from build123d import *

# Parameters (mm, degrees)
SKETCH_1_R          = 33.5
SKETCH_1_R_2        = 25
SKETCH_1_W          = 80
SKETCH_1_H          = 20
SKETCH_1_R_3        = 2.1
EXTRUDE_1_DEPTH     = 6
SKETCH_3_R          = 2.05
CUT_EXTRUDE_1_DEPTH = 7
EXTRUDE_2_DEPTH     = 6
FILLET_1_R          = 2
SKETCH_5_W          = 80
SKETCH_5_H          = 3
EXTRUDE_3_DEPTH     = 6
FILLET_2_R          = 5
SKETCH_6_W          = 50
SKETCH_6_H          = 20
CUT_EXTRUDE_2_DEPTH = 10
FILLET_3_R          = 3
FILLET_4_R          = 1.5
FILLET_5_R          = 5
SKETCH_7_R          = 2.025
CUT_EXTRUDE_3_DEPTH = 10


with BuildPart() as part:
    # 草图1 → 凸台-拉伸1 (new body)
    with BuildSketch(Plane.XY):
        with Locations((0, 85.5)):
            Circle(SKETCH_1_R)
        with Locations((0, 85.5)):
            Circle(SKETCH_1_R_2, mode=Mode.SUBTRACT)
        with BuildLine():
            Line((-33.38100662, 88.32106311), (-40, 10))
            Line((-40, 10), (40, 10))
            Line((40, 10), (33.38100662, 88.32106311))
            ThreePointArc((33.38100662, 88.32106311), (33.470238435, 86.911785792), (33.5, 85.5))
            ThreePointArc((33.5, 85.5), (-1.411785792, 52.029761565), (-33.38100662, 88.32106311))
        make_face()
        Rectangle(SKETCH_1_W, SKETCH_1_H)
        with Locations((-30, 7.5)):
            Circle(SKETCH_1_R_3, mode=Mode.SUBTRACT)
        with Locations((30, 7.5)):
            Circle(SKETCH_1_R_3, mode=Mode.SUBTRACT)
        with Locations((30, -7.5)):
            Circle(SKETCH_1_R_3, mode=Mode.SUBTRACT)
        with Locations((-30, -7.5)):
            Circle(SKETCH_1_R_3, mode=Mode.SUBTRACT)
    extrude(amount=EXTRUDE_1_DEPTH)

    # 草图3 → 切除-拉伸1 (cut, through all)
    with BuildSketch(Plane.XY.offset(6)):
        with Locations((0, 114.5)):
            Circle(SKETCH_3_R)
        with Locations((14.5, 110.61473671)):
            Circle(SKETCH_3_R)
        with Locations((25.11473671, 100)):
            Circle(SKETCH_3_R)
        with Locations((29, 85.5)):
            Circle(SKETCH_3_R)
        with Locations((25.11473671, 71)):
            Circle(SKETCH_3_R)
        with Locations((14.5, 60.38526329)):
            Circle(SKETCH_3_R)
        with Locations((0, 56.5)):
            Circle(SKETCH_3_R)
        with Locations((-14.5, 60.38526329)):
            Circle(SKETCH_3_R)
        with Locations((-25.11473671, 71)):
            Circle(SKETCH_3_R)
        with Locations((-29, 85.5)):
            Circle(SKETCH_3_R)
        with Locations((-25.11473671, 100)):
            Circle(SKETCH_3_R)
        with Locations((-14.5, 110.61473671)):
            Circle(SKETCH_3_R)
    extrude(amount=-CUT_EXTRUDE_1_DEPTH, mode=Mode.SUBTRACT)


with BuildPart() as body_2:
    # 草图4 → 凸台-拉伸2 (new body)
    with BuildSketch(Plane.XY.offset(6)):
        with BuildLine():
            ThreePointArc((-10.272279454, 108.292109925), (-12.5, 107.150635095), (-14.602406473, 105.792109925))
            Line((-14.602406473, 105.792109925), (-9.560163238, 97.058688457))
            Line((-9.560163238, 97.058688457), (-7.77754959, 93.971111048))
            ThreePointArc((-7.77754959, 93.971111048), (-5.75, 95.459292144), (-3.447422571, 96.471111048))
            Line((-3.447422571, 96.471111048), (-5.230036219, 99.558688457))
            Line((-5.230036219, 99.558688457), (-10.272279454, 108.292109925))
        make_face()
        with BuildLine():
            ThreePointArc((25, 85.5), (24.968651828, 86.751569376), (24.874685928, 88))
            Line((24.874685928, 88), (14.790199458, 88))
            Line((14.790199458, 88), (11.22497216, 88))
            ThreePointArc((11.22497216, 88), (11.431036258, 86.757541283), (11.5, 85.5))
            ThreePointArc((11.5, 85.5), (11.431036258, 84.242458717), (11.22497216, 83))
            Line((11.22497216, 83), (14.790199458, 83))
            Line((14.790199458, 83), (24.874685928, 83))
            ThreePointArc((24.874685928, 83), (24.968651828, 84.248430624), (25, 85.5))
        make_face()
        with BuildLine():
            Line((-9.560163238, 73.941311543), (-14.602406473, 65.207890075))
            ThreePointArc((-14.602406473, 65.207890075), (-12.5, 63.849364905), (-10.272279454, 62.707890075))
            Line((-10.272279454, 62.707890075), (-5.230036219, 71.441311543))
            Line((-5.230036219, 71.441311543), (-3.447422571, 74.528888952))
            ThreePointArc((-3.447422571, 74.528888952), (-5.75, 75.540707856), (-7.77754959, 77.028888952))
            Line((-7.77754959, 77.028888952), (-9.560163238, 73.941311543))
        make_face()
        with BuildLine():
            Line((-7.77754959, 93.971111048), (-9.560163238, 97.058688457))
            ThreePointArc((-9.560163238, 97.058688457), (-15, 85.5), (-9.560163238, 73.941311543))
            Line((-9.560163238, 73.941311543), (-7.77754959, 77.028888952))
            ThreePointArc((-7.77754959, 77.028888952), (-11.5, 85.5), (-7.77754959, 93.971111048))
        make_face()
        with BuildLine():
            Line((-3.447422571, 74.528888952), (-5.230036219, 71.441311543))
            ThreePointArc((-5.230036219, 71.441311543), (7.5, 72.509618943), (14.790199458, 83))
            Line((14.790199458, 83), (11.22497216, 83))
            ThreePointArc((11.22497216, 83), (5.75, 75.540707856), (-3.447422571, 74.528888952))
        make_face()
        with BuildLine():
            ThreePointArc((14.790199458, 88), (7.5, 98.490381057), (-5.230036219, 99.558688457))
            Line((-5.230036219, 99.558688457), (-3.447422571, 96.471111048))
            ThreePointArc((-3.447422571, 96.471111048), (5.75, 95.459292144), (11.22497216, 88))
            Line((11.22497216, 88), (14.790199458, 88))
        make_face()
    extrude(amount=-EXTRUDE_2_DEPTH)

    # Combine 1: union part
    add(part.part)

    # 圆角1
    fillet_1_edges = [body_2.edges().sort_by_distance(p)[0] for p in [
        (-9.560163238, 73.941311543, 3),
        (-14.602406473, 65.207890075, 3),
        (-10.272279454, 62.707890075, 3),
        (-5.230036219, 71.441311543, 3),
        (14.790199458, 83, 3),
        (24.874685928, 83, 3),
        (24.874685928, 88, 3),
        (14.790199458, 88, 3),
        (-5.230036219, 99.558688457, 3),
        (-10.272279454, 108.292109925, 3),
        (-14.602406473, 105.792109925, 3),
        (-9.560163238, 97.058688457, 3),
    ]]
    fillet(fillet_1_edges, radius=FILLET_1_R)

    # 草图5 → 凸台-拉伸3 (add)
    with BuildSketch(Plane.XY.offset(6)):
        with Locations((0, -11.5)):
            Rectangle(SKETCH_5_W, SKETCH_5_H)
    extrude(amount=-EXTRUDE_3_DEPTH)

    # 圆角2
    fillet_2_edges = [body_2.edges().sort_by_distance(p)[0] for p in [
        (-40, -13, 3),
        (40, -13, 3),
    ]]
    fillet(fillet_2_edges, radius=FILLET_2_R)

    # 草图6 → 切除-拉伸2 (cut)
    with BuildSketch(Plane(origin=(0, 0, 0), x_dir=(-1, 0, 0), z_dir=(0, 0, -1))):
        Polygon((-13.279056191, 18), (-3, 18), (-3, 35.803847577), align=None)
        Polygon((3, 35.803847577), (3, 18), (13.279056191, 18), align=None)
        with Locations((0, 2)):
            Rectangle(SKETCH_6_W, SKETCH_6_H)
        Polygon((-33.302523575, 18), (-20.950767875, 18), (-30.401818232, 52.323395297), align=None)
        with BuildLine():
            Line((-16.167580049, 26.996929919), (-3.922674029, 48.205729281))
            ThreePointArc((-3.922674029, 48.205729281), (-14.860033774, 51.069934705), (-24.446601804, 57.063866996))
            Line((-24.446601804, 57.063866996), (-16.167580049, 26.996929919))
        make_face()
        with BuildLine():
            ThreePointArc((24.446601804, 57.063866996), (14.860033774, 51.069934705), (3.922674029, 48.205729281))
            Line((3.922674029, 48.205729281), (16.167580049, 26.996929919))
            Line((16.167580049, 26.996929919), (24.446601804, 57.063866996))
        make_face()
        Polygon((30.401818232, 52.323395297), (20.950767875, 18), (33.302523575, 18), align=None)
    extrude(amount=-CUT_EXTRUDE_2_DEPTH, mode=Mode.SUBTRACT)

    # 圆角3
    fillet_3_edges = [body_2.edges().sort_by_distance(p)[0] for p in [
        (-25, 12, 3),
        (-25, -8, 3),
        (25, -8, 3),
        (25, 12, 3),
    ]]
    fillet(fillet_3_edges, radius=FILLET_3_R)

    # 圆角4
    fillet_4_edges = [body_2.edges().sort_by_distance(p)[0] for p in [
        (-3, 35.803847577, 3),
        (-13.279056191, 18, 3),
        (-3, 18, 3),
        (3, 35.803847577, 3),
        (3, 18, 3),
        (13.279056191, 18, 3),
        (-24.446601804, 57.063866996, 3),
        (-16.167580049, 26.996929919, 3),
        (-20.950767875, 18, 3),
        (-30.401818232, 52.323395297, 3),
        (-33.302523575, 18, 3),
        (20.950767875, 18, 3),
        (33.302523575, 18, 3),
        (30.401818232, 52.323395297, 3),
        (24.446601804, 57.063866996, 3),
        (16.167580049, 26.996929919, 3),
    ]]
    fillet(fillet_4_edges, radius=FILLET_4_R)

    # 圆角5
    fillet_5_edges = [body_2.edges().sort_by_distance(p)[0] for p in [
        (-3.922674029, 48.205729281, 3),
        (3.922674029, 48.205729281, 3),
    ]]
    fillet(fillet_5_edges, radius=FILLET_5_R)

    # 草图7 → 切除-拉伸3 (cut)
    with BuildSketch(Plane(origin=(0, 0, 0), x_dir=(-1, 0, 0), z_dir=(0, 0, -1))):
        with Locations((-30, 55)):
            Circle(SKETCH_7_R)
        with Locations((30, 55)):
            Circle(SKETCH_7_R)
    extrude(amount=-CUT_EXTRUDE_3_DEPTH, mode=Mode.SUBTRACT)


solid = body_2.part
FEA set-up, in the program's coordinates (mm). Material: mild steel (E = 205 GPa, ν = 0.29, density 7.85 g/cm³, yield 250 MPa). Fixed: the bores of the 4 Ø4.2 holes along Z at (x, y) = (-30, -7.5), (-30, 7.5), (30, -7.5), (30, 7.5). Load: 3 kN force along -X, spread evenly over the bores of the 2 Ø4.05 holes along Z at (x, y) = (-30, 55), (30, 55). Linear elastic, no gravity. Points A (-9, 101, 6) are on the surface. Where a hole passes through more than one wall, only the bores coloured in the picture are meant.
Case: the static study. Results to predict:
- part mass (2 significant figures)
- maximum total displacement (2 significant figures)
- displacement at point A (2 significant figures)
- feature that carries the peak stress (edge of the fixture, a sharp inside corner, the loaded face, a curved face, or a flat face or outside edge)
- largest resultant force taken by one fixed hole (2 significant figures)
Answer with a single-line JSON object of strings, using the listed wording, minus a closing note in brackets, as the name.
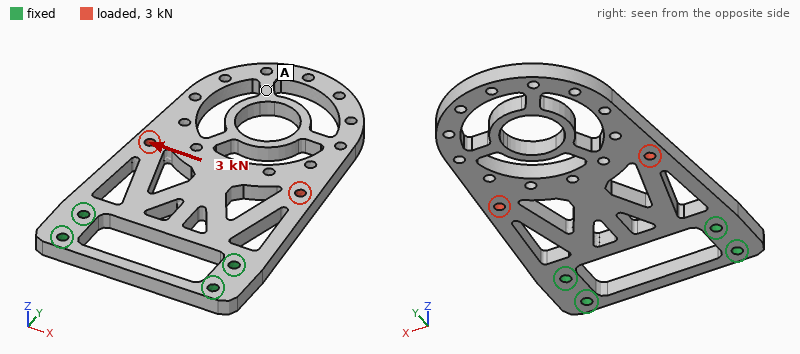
{"part mass": "250 g", "maximum total displacement": "29 µm", "displacement at point A": "26 µm", "feature that carries the peak stress": "a curved face", "largest resultant force taken by one fixed hole": "2.5 kN"}
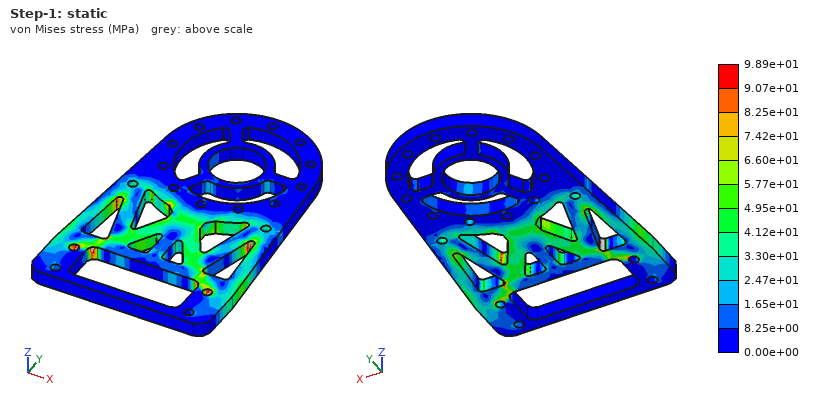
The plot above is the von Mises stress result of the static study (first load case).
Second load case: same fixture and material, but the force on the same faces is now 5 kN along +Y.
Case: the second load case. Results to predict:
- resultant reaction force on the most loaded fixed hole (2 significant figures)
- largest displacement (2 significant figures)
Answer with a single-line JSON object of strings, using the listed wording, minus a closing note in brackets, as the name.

{"resultant reaction force on the most loaded fixed hole": "2.2 kN", "largest displacement": "10 µm"}
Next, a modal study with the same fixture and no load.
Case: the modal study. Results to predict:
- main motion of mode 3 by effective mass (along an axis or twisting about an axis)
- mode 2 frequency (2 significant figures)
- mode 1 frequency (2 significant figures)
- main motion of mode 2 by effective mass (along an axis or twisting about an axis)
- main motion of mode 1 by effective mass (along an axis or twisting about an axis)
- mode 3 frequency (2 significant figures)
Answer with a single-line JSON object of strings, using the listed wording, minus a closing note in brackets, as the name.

{"main motion of mode 3 by effective mass": "along Z", "mode 2 frequency": "1400 Hz", "mode 1 frequency": "390 Hz", "main motion of mode 2 by effective mass": "twisting about Y", "main motion of mode 1 by effective mass": "along Z", "mode 3 frequency": "2000 Hz"}
